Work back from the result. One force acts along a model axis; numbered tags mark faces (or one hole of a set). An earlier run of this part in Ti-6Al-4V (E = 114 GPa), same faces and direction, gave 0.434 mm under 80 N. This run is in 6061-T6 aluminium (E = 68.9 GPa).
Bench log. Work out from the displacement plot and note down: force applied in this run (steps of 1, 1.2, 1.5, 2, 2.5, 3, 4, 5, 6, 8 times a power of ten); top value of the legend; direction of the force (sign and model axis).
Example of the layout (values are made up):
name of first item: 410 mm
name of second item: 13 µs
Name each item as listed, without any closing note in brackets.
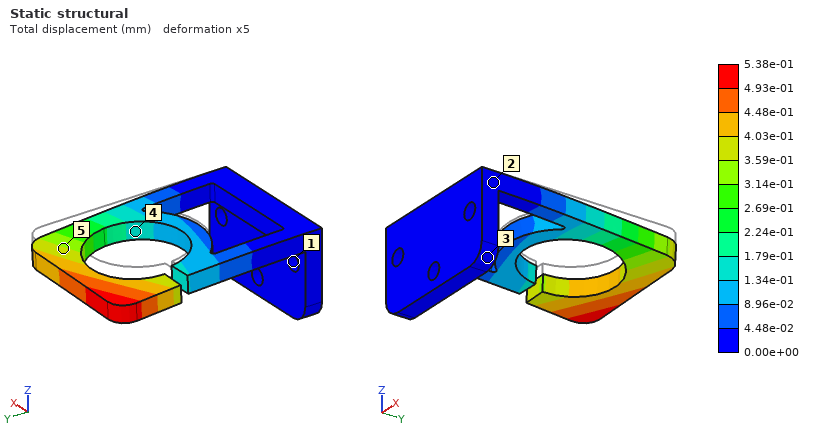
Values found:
force applied in this run: 60 N
top value of the legend: 5.38e-01 mm
direction of the force: -Z
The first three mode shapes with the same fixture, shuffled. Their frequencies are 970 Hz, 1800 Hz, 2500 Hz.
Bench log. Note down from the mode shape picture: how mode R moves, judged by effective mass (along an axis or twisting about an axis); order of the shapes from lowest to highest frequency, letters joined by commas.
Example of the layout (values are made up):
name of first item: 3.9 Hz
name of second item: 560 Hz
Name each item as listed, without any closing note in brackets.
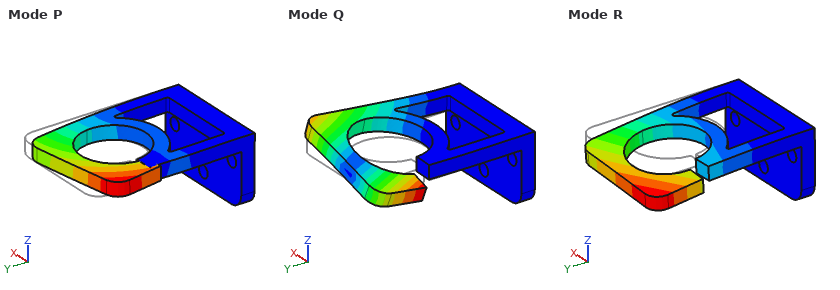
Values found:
how mode R moves, judged by effective mass: along Z
order of the shapes from lowest to highest frequency, letters joined by commas: R, P, Q
